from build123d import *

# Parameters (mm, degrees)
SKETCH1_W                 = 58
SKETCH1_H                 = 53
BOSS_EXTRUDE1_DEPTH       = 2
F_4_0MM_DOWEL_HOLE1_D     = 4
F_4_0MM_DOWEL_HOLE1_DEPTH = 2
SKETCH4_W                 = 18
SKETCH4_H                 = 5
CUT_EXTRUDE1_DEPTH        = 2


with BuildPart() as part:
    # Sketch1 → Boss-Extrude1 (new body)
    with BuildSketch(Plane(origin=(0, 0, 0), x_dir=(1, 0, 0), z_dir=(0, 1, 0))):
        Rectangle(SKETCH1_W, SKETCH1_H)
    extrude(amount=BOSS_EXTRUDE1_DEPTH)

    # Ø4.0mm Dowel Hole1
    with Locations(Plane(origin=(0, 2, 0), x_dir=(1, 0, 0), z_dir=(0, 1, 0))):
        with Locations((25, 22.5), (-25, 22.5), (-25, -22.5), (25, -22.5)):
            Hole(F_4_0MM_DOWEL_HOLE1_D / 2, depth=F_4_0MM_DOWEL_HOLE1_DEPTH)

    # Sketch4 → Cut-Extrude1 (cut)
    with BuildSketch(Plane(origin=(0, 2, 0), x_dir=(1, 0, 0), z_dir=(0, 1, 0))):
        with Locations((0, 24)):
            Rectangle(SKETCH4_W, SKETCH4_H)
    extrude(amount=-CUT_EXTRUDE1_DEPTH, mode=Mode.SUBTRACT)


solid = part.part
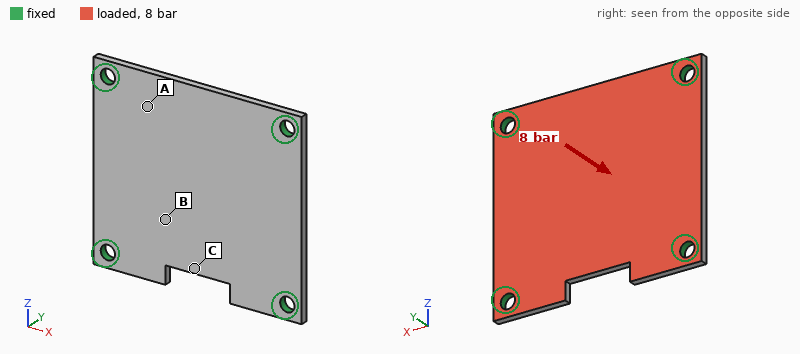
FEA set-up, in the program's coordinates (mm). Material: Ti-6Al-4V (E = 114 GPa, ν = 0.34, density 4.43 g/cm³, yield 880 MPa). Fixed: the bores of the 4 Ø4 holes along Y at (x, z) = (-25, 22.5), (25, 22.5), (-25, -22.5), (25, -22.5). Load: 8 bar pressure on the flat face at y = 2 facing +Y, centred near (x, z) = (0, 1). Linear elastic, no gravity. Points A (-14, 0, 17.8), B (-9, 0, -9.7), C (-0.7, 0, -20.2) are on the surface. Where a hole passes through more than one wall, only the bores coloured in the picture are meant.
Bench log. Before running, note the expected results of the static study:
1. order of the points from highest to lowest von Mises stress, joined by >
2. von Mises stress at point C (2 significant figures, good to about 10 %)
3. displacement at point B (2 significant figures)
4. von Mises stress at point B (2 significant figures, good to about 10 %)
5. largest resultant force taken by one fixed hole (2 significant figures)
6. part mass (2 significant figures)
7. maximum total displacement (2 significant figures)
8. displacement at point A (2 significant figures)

C > B > A
170 MPa
0.25 mm
110 MPa
600 N
26 g
0.32 mm
0.13 mm
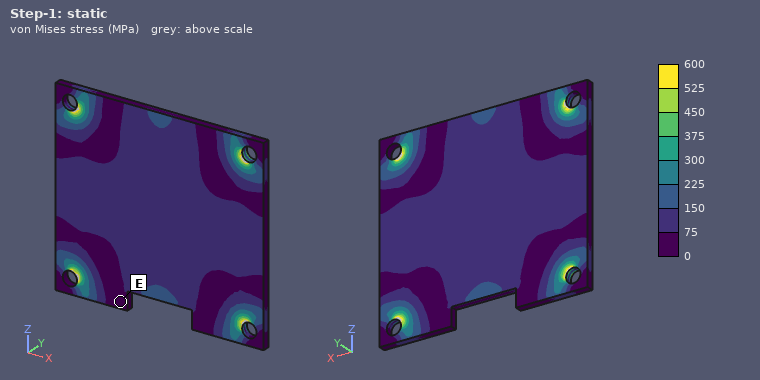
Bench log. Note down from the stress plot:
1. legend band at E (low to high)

0 to 75 MPa
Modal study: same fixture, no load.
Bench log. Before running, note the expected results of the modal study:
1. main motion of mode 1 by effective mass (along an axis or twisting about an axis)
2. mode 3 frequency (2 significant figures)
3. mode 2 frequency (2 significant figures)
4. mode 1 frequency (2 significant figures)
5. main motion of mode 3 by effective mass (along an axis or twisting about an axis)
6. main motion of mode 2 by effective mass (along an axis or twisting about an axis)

along Y
5900 Hz
5300 Hz
3200 Hz
twisting about Z
twisting about X
